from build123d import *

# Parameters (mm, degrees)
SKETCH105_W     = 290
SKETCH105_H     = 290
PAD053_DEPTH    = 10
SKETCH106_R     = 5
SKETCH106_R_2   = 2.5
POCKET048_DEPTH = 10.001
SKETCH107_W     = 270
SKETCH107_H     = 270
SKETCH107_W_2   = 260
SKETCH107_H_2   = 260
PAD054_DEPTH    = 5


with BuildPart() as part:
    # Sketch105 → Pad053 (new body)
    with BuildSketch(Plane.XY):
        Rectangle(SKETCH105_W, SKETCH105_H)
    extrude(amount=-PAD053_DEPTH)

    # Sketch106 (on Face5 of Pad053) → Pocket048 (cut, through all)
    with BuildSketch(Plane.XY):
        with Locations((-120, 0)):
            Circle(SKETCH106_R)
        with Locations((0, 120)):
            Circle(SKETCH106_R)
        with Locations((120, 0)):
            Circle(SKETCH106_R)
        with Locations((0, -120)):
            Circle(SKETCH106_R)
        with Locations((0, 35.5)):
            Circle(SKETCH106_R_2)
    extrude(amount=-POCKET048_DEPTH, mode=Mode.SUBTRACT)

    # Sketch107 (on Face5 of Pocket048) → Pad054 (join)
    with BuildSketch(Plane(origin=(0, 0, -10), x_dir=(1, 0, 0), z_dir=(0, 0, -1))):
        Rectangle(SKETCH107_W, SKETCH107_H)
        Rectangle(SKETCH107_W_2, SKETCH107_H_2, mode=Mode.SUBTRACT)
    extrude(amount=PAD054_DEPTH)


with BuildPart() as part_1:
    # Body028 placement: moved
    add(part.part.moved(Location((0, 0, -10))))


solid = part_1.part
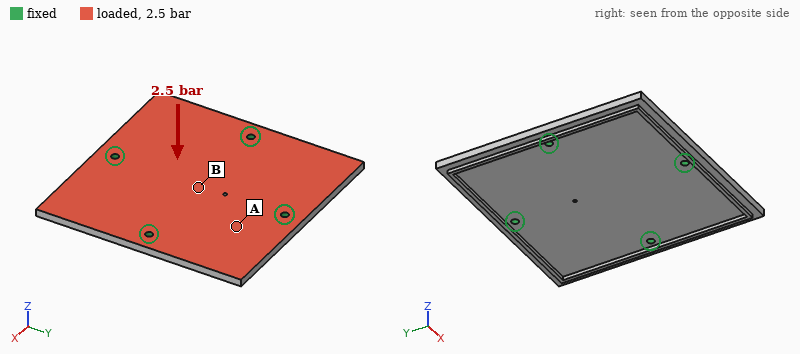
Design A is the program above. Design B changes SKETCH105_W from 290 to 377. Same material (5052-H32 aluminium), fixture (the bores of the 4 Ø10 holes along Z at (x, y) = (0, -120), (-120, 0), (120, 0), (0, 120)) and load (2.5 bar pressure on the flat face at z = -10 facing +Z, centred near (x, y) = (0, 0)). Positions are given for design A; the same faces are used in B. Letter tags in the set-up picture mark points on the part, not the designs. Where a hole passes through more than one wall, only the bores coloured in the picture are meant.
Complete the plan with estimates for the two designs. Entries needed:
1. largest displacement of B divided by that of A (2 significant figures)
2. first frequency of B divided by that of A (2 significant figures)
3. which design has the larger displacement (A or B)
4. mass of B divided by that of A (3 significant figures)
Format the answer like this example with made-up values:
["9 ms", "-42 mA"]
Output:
["2.1", "0.70", "B", "1.29"]
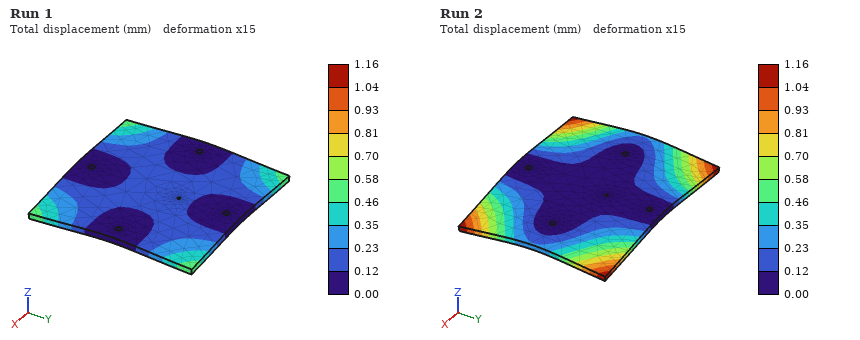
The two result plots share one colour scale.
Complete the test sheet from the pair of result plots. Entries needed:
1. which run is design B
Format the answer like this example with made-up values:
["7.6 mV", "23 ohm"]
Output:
["Run 2"]
